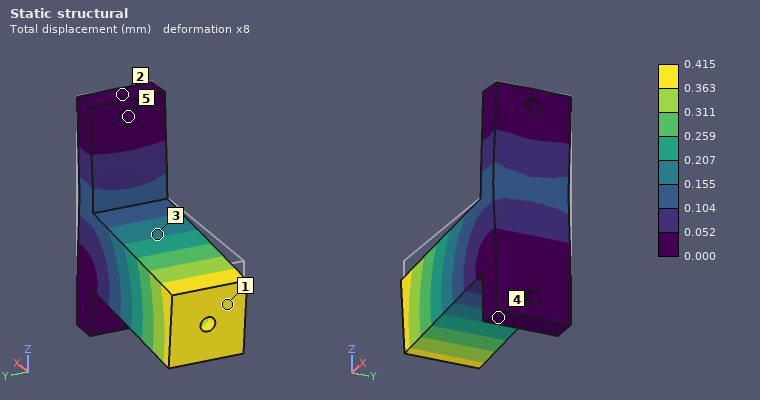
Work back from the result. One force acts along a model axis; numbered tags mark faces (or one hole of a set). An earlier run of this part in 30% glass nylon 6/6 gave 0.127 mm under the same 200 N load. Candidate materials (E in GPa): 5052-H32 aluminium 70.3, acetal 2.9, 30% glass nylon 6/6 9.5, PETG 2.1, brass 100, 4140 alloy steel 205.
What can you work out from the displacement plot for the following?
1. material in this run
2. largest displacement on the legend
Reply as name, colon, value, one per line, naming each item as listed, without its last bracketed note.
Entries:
material in this run: acetal
largest displacement on the legend: 0.415 mm
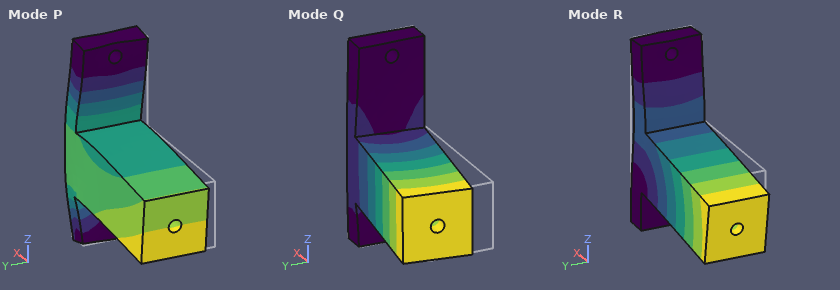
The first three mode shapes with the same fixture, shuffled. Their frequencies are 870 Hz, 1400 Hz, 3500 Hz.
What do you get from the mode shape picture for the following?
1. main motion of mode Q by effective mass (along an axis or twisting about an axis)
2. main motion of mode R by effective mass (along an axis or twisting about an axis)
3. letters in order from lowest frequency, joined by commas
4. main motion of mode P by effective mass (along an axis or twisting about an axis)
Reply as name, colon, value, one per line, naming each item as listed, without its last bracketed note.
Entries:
main motion of mode Q by effective mass: along Y
main motion of mode R by effective mass: along Z
letters in order from lowest frequency, joined by commas: Q, R, P
main motion of mode P by effective mass: along X
